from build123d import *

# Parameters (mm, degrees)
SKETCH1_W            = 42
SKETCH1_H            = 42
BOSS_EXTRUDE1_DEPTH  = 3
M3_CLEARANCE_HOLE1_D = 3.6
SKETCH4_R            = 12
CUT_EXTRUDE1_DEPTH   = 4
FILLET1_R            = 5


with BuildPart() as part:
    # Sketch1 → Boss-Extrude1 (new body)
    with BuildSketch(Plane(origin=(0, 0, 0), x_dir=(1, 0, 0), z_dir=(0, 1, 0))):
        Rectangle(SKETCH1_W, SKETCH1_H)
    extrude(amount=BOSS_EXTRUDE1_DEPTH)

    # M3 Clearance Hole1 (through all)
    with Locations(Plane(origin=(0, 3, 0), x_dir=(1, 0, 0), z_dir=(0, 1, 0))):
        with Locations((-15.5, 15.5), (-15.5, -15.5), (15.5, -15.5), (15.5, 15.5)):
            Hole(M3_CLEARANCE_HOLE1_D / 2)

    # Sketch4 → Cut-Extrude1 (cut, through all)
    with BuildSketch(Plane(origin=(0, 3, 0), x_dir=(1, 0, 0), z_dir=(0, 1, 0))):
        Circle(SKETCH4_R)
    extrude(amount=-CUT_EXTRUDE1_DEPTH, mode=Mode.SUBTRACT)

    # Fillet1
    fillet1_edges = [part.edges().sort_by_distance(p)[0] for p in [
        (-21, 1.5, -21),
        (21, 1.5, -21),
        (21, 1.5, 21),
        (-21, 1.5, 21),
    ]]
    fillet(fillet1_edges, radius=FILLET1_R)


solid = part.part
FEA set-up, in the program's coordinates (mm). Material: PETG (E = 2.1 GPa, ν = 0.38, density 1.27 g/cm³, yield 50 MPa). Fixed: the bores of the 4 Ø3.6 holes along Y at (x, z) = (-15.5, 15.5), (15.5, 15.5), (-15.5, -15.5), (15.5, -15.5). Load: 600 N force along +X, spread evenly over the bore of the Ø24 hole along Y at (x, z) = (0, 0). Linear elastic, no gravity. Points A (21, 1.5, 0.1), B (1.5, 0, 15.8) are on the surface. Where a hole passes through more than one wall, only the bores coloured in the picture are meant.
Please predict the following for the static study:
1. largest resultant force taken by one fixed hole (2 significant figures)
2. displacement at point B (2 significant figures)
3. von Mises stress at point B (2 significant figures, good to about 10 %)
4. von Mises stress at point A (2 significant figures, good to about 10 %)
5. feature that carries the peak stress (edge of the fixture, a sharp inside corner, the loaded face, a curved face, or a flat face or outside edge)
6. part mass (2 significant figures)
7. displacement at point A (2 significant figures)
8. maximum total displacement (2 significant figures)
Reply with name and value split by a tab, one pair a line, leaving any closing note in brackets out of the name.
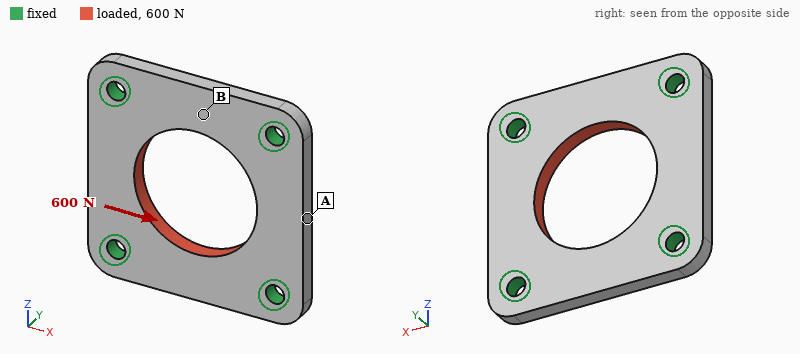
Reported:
largest resultant force taken by one fixed hole	150 N
displacement at point B	17 µm
von Mises stress at point B	3.8 MPa
von Mises stress at point A	6.4 MPa
feature that carries the peak stress	edge of the fixture
part mass	4.8 g
displacement at point A	58 µm
maximum total displacement	65 µm
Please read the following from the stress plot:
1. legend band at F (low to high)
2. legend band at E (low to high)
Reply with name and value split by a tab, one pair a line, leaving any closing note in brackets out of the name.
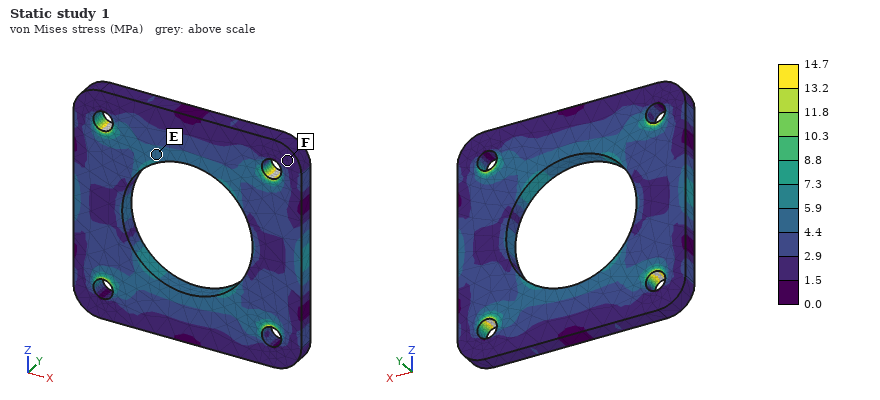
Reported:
legend band at F	1.5 to 2.9 MPa
legend band at E	4.4 to 5.9 MPa
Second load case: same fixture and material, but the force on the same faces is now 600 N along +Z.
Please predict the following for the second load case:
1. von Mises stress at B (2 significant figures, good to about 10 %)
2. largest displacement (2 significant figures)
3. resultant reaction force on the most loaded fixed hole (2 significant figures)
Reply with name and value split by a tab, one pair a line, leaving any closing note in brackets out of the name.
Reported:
von Mises stress at B	2.2 MPa
largest displacement	65 µm
resultant reaction force on the most loaded fixed hole	150 N
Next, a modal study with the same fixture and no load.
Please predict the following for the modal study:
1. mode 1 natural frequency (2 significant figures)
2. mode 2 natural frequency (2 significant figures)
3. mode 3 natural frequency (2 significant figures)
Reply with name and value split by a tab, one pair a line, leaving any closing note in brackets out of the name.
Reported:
mode 1 natural frequency	4400 Hz
mode 2 natural frequency	4600 Hz
mode 3 natural frequency	4600 Hz
